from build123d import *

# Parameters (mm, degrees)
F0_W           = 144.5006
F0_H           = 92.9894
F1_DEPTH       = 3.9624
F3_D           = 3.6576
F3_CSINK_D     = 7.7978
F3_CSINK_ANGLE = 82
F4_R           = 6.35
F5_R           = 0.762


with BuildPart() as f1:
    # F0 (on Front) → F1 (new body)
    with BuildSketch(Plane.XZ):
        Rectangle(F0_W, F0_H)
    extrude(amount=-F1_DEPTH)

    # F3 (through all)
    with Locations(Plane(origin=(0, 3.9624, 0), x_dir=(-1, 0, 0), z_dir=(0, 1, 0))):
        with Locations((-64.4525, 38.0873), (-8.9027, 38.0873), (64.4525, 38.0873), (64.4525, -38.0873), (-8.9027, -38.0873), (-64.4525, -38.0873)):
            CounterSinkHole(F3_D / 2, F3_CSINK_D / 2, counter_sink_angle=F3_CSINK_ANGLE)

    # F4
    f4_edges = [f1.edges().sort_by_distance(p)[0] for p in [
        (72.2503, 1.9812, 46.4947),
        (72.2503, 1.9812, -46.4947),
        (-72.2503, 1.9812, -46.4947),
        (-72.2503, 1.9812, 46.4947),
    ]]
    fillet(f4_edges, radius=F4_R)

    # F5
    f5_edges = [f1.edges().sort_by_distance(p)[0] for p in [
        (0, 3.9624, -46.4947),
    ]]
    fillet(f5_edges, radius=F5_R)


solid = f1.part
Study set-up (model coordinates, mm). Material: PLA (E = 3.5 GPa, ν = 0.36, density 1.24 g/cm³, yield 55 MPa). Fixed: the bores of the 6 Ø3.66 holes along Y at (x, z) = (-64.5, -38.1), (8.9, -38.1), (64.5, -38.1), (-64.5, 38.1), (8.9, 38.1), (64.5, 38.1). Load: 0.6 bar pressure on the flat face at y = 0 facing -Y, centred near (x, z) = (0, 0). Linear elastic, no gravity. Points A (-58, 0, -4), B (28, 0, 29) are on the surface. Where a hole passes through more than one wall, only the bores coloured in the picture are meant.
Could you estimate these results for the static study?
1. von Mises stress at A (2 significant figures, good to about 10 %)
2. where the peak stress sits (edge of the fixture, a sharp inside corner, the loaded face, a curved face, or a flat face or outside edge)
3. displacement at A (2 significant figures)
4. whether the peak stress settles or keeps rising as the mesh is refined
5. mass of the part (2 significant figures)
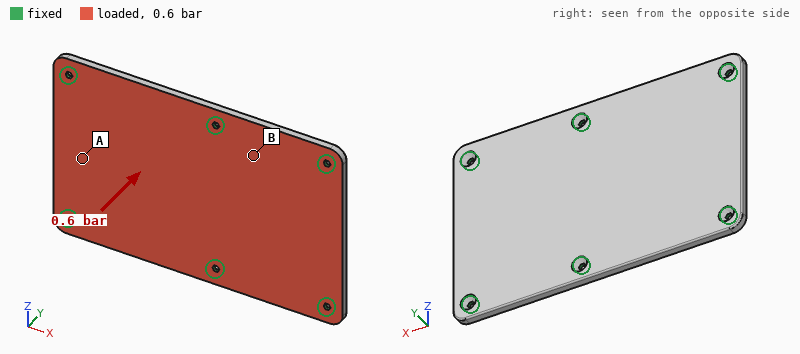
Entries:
7.2 MPa
edge of the fixture
0.67 mm
keeps rising
65 g
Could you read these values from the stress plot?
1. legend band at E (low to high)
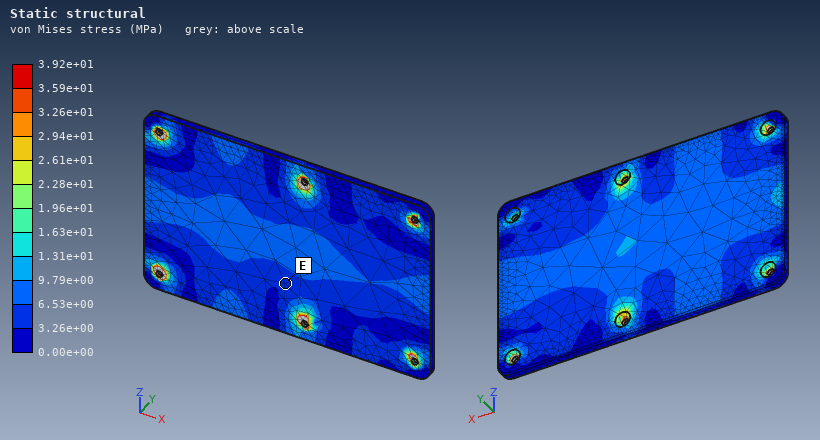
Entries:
3.26e+00 to 6.53e+00 MPa
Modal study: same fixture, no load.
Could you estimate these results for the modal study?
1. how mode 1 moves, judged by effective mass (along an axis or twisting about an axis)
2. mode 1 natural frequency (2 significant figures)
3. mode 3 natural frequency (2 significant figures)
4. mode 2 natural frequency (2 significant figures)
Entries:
along Y
700 Hz
1200 Hz
870 Hz
